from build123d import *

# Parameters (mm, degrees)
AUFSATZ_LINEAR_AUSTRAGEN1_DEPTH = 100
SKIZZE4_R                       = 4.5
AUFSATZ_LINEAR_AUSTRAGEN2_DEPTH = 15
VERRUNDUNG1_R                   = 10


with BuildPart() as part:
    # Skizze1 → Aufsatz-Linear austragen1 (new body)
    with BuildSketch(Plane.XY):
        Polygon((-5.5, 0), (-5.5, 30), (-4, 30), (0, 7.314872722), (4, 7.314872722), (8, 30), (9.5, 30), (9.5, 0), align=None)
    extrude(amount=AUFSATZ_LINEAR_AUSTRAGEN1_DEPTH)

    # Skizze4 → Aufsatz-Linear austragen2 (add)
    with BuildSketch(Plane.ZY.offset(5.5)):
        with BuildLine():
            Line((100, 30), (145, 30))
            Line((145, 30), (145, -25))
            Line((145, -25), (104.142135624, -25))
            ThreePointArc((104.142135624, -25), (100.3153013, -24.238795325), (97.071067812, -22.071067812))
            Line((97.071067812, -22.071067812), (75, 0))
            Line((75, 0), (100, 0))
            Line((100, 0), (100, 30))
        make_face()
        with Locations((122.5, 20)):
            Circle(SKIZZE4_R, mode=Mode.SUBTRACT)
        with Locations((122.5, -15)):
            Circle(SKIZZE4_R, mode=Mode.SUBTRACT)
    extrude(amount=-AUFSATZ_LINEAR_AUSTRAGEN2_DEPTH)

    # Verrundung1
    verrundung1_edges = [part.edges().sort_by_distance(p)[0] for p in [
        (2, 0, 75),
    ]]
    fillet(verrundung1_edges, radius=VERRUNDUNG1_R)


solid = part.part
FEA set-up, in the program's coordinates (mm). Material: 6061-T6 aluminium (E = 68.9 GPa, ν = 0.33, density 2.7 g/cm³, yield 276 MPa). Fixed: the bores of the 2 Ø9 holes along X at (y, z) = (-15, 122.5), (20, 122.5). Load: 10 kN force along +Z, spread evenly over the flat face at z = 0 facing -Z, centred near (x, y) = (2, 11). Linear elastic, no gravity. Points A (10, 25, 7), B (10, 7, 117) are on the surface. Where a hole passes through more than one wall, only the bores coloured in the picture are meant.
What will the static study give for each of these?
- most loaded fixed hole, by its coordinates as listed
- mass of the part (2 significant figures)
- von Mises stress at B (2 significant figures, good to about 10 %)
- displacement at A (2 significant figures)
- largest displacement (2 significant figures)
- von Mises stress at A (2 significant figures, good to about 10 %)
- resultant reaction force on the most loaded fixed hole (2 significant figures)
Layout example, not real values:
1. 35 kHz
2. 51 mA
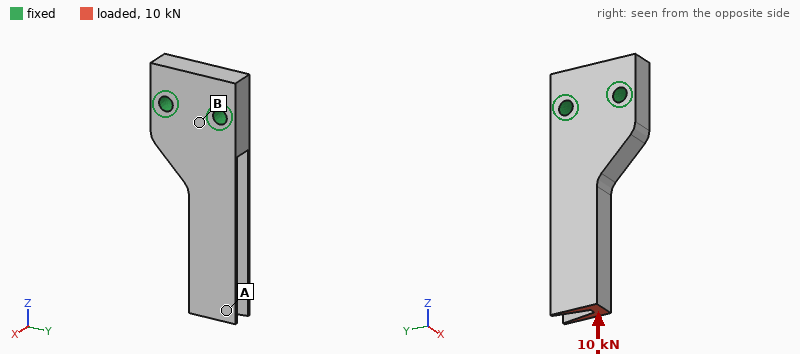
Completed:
1. (20, 122.5)
2. 180 g
3. 8.6 MPa
4. 79 µm
5. 87 µm
6. 37 MPa
7. 7.4 kN
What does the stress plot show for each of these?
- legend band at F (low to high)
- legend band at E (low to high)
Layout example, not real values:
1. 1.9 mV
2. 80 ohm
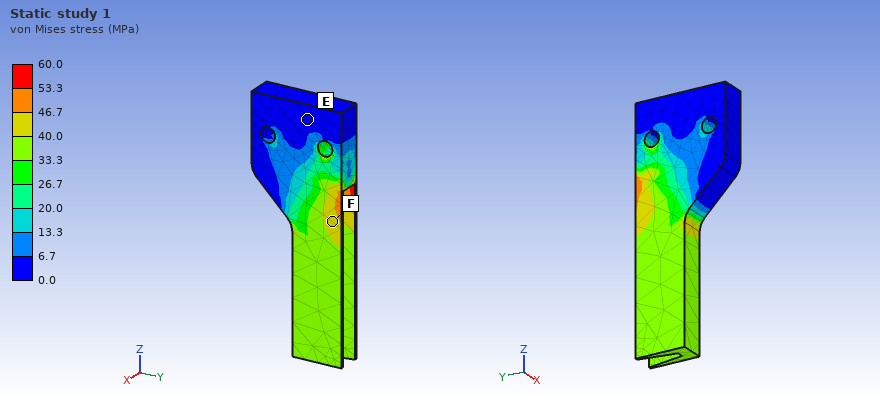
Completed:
1. 40.0 to 46.7 MPa
2. 0.0 to 6.7 MPa
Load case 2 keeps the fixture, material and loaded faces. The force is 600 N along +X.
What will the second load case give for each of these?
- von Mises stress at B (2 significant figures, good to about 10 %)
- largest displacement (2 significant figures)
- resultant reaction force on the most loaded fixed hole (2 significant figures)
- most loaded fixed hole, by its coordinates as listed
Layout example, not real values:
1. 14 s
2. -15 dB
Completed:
1. 24 MPa
2. 0.82 mm
3. 420 N
4. (20, 122.5)
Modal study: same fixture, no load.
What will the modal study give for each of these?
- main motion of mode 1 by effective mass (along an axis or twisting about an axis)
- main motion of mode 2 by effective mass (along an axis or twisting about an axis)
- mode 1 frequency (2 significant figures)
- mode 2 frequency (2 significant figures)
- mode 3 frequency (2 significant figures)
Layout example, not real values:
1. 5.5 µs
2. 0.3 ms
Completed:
1. along X
2. along Y
3. 1100 Hz
4. 2400 Hz
5. 3500 Hz
